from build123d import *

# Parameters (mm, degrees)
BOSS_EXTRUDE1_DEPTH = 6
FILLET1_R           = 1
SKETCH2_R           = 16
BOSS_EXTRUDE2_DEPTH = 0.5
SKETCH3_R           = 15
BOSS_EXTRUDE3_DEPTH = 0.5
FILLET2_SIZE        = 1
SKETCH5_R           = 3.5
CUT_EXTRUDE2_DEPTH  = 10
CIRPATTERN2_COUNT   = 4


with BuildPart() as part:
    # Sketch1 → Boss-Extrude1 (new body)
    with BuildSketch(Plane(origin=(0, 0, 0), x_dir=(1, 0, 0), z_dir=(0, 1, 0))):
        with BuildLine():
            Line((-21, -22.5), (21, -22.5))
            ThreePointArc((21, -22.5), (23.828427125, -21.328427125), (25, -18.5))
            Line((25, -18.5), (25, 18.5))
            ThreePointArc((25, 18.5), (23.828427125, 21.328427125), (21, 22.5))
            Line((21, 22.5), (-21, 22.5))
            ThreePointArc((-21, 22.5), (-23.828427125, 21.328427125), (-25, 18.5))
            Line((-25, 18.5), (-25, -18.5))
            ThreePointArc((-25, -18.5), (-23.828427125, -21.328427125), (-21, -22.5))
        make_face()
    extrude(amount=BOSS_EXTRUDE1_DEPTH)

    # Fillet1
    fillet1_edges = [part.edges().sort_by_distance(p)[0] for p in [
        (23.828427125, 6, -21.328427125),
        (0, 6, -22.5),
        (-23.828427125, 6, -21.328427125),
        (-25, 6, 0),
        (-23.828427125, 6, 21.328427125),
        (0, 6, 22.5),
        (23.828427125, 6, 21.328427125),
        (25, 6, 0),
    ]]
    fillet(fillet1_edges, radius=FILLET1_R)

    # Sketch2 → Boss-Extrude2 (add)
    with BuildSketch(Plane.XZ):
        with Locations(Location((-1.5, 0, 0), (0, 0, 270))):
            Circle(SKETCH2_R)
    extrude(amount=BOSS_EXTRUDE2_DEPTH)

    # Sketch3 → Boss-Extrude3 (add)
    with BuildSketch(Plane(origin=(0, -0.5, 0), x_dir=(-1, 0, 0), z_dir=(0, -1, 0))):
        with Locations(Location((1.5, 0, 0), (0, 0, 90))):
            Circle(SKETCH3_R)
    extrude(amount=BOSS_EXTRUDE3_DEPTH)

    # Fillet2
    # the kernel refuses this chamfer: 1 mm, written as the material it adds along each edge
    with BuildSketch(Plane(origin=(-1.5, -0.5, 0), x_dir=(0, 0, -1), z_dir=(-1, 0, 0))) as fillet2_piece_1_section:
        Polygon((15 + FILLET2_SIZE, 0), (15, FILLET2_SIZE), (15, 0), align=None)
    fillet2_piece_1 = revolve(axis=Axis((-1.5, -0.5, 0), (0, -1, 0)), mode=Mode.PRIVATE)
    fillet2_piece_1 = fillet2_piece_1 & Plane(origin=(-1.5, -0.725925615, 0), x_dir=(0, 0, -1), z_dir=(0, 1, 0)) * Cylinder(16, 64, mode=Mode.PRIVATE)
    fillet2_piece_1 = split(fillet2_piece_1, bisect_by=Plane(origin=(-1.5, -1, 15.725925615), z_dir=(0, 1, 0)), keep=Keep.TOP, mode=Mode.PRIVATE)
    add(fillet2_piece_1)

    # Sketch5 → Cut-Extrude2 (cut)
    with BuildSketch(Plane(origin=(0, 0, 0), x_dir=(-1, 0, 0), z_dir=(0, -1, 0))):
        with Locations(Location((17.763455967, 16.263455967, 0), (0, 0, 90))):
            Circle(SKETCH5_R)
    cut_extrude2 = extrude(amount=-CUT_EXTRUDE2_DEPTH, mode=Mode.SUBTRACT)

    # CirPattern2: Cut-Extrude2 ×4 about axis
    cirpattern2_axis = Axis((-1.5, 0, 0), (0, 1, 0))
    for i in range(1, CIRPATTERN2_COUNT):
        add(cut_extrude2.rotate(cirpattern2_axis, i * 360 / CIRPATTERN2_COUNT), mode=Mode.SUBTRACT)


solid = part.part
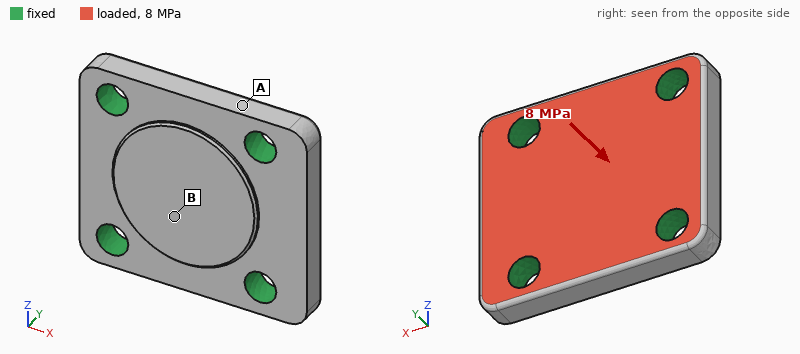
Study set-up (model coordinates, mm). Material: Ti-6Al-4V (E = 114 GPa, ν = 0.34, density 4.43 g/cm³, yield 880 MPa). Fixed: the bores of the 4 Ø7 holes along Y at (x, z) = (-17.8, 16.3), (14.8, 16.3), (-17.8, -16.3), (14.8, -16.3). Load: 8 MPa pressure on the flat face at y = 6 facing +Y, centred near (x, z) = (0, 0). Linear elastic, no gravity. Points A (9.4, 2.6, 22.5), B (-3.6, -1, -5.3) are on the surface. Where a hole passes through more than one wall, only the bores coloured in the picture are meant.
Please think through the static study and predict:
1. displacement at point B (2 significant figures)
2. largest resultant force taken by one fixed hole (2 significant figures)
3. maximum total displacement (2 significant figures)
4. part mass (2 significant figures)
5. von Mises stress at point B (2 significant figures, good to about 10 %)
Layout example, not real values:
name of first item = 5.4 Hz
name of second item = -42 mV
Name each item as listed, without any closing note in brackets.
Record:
displacement at point B = 16 µm
largest resultant force taken by one fixed hole = 4.1 kN
maximum total displacement = 18 µm
part mass = 59 g
von Mises stress at point B = 46 MPa
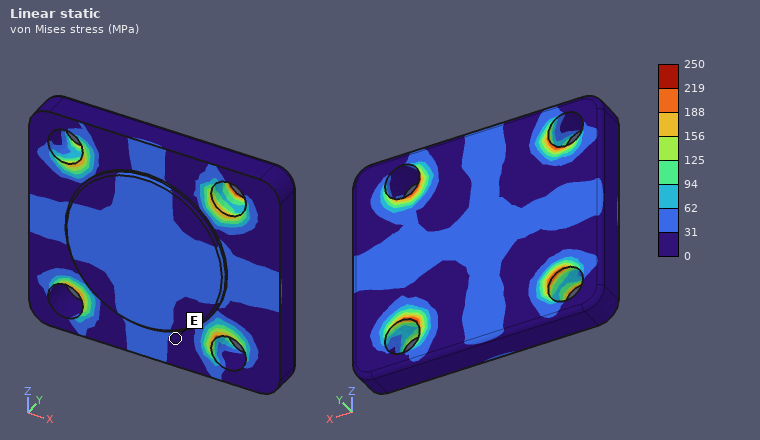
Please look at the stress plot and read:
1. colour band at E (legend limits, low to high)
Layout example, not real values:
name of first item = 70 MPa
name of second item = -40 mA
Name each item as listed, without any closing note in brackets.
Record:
colour band at E = 0 to 31 MPa
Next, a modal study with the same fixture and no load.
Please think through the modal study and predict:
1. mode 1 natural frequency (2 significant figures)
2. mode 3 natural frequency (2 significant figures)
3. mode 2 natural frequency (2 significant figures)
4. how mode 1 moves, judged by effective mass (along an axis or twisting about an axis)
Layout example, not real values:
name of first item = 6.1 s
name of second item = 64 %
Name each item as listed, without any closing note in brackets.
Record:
mode 1 natural frequency = 23 kHz
mode 3 natural frequency = 34 kHz
mode 2 natural frequency = 29 kHz
how mode 1 moves, judged by effective mass = along Y
